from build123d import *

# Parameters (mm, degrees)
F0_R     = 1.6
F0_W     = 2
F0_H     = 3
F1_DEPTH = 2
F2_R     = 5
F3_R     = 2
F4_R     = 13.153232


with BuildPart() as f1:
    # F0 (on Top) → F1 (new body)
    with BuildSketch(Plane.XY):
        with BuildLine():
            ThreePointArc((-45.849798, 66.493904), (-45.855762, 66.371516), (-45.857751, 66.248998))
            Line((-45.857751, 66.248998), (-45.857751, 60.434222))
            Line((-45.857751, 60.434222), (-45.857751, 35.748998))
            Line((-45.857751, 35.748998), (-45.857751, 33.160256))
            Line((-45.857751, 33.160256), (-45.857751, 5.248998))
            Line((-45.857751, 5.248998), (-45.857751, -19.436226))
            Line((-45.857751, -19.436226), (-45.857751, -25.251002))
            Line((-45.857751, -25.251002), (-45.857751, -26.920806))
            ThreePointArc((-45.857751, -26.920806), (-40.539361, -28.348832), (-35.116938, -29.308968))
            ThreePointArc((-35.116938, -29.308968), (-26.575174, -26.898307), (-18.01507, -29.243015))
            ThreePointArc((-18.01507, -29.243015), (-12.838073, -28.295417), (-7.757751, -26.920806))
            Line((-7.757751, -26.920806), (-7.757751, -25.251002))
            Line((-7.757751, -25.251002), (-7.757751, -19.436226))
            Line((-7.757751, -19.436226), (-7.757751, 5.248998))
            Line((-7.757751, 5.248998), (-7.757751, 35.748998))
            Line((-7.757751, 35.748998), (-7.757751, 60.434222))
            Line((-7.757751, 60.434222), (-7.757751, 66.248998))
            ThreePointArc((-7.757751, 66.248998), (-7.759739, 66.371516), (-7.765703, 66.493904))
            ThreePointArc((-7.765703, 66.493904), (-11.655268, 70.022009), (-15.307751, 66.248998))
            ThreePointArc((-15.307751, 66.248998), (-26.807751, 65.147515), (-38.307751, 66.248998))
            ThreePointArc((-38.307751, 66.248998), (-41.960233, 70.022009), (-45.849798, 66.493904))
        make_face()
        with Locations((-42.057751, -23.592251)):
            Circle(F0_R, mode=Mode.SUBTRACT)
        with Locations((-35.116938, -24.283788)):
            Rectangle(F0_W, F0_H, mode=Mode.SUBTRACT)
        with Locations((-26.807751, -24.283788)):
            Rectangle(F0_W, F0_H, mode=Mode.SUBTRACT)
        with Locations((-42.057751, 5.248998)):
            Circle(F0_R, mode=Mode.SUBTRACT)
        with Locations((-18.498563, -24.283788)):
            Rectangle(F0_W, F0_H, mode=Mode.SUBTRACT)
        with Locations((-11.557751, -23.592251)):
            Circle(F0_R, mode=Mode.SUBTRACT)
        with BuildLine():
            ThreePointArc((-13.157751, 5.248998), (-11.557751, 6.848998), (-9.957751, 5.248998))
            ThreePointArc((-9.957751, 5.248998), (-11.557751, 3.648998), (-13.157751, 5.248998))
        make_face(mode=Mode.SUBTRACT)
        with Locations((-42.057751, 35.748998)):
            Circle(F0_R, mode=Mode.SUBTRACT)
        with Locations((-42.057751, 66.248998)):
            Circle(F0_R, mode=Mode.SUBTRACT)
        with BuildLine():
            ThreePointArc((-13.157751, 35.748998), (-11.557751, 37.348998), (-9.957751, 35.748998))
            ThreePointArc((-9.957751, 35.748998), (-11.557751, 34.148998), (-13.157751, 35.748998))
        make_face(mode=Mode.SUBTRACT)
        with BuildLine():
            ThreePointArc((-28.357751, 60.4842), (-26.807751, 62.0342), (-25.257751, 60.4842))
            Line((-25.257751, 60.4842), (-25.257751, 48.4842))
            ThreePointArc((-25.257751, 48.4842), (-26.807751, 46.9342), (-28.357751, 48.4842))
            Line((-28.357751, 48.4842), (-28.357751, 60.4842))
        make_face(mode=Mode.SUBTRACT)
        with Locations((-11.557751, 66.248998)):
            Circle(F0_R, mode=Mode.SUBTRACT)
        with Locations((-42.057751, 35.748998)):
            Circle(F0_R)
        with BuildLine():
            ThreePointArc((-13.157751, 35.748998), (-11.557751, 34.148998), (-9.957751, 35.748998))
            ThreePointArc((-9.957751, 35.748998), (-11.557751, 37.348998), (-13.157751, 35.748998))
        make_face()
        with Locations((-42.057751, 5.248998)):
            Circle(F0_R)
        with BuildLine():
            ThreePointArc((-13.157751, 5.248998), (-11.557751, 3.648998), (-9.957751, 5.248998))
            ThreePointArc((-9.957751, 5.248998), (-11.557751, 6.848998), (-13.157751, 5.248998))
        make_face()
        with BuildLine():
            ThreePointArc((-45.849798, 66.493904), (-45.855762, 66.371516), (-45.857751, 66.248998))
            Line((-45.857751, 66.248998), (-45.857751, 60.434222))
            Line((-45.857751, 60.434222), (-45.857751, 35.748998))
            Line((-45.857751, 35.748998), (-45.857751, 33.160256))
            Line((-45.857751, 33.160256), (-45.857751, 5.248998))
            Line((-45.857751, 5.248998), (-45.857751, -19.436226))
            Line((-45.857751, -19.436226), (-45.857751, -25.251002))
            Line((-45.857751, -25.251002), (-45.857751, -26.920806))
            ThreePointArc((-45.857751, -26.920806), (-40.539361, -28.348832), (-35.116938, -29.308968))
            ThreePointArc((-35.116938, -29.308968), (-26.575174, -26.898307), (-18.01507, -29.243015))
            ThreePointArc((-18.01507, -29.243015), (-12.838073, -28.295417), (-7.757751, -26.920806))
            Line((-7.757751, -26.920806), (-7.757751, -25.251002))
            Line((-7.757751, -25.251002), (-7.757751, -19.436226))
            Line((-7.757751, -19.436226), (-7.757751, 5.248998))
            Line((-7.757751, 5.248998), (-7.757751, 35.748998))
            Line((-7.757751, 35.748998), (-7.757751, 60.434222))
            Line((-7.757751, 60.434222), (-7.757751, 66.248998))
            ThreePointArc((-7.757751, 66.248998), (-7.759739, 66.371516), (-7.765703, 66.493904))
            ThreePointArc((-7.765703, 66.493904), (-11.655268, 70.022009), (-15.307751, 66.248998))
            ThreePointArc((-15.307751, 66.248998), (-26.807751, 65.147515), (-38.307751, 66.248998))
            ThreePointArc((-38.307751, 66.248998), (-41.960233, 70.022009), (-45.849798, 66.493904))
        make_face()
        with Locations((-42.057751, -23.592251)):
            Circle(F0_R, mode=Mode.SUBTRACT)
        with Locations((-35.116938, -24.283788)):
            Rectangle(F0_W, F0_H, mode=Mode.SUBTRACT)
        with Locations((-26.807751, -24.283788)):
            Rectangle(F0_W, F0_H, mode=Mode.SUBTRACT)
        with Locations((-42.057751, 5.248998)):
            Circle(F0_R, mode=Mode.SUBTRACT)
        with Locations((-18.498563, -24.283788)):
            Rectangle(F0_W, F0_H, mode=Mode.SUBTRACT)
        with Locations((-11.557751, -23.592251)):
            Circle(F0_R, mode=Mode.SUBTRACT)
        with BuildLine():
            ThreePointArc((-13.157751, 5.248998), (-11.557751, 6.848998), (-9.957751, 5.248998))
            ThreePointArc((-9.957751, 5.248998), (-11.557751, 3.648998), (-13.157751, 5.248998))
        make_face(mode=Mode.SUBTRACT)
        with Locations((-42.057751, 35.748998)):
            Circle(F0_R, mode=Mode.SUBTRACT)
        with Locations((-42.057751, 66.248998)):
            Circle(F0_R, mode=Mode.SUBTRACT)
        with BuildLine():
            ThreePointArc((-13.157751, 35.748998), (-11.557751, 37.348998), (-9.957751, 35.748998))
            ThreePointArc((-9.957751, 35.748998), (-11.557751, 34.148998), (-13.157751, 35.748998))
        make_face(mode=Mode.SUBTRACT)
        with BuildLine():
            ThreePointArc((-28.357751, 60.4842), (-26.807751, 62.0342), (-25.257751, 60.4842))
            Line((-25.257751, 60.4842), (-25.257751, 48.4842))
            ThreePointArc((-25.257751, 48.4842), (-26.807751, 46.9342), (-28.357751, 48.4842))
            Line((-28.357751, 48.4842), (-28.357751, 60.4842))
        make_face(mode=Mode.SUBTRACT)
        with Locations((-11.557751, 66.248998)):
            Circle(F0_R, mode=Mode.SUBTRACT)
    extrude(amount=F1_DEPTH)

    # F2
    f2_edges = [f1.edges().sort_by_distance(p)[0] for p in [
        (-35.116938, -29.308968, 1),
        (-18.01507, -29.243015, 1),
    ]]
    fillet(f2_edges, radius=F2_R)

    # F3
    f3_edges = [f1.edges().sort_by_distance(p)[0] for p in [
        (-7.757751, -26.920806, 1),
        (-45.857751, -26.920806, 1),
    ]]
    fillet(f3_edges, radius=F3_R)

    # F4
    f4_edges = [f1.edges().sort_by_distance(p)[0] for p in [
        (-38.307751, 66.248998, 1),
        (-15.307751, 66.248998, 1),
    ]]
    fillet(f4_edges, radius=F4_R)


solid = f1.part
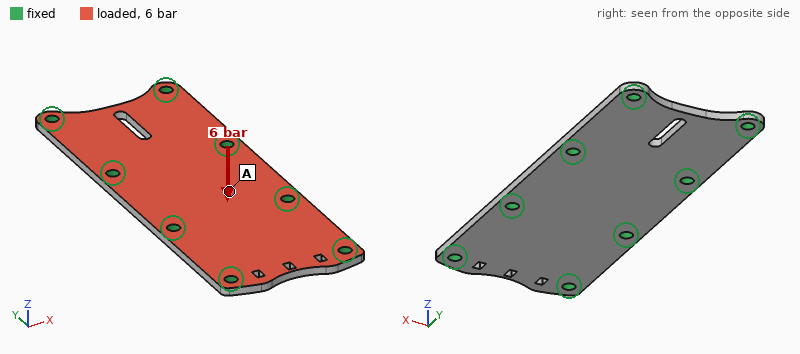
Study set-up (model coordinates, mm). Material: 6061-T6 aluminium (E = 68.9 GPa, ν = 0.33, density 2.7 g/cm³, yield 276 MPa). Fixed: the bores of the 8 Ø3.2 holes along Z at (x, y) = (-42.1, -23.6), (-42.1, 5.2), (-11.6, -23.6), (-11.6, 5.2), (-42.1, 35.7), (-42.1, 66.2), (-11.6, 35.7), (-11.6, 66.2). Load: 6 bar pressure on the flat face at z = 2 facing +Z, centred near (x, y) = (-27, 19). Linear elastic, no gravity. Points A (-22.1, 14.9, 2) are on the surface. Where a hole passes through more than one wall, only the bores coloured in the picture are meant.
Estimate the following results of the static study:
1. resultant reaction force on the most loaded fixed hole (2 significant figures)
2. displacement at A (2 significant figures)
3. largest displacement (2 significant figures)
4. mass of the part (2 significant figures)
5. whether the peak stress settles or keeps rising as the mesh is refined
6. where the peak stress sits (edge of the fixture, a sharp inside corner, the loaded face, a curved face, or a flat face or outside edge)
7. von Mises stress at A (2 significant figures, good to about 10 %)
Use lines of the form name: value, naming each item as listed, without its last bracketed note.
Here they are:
resultant reaction force on the most loaded fixed hole: 350 N
displacement at A: 48 µm
largest displacement: 77 µm
mass of the part: 19 g
whether the peak stress settles or keeps rising as the mesh is refined: keeps rising
where the peak stress sits: edge of the fixture
von Mises stress at A: 28 MPa
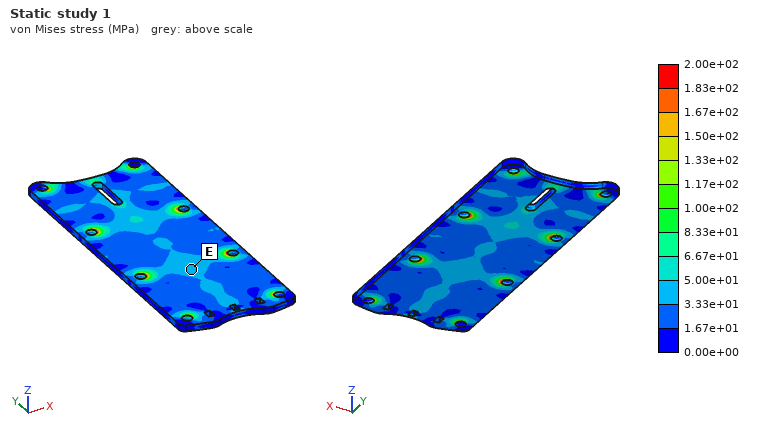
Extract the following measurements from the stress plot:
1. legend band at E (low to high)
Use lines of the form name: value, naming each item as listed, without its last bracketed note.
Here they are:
legend band at E: 3.33e+01 to 5.00e+01 MPa
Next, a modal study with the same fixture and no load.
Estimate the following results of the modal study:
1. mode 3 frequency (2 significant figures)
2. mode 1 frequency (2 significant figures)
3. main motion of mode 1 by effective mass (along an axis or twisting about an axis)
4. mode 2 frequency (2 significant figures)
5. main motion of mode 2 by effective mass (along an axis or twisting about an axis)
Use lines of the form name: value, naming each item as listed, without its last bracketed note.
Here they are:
mode 3 frequency: 8900 Hz
mode 1 frequency: 7800 Hz
main motion of mode 1 by effective mass: along Z
mode 2 frequency: 8500 Hz
main motion of mode 2 by effective mass: along Z
